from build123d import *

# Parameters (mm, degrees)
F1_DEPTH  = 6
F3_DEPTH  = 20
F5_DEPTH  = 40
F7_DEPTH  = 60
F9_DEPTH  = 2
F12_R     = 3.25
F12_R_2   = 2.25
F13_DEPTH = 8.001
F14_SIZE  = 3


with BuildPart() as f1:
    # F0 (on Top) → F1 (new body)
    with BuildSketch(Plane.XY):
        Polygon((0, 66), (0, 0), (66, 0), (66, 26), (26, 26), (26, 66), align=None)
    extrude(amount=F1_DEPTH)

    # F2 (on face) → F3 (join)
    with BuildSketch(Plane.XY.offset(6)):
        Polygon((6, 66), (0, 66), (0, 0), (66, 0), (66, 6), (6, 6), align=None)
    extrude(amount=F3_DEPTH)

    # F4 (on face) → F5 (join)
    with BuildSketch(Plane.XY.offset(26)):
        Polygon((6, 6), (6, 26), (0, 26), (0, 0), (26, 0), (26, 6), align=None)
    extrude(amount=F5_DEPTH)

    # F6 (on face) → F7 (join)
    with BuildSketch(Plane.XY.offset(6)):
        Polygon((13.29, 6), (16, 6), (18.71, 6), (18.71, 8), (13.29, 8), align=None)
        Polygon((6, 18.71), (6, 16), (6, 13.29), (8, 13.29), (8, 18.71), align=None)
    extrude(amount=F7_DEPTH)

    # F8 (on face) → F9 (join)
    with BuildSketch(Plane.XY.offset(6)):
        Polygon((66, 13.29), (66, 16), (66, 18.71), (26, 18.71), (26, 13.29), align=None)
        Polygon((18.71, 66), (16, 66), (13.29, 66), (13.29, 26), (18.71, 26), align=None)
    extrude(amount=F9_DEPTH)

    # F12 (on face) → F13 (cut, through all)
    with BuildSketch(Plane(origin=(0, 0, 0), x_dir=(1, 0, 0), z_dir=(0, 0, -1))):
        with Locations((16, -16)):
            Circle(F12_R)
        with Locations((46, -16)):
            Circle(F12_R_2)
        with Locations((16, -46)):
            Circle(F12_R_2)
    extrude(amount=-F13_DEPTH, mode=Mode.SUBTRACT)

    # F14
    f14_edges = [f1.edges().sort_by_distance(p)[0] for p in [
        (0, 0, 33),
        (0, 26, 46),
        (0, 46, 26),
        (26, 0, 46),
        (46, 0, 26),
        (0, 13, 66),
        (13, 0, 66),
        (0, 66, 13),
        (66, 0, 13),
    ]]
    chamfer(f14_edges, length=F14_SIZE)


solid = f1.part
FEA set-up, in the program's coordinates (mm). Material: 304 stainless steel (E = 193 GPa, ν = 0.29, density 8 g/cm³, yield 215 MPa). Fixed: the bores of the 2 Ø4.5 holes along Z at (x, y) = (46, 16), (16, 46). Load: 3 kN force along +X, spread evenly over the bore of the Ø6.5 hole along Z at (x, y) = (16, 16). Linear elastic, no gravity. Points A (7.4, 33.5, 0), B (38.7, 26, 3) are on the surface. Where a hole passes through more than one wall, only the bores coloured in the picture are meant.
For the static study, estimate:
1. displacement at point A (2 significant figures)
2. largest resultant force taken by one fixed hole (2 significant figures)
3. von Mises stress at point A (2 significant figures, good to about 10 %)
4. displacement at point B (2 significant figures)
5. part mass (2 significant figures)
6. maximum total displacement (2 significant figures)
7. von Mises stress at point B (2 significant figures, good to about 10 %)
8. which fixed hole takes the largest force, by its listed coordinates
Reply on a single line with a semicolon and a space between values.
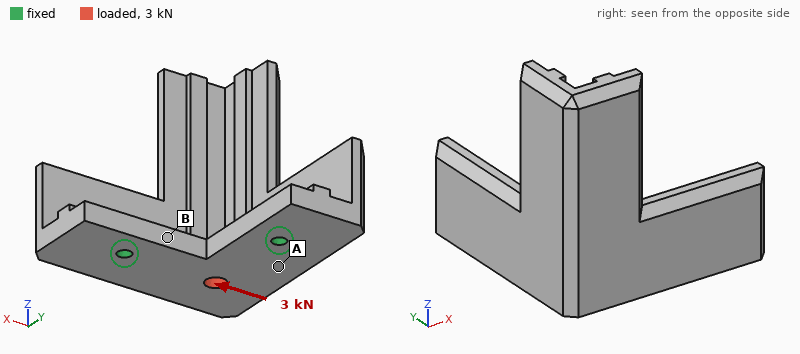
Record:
1.9 µm; 2.6 kN; 5.4 MPa; 0.84 µm; 340 g; 5.1 µm; 15 MPa; (46, 16)
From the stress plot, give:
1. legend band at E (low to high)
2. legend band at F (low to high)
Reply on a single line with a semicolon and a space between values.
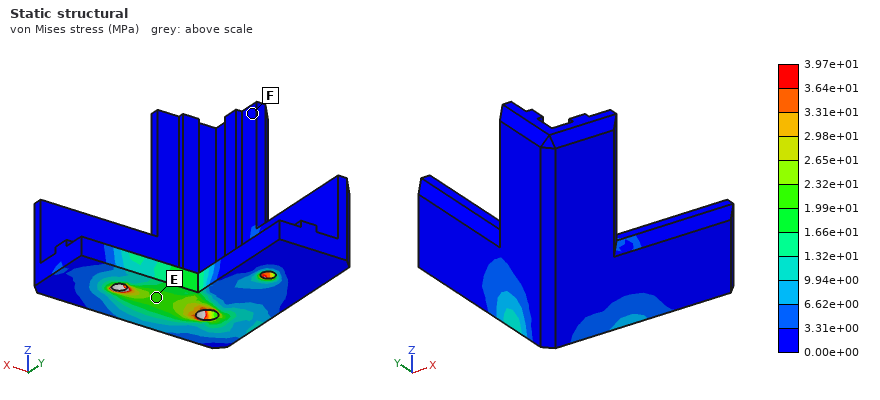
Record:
1.99e+01 to 2.32e+01 MPa; 0.00e+00 to 3.31e+00 MPa
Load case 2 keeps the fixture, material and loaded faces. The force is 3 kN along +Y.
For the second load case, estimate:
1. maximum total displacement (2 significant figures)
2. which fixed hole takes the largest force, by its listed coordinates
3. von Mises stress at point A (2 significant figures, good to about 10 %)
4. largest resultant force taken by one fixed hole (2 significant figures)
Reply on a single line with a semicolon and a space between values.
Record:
5.1 µm; (16, 46); 15 MPa; 2.6 kN
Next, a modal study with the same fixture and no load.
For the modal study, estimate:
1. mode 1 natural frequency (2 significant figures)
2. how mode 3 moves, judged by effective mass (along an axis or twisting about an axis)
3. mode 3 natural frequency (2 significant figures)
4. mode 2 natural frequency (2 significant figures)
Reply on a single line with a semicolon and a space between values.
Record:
1300 Hz; along Z; 4900 Hz; 2900 Hz
